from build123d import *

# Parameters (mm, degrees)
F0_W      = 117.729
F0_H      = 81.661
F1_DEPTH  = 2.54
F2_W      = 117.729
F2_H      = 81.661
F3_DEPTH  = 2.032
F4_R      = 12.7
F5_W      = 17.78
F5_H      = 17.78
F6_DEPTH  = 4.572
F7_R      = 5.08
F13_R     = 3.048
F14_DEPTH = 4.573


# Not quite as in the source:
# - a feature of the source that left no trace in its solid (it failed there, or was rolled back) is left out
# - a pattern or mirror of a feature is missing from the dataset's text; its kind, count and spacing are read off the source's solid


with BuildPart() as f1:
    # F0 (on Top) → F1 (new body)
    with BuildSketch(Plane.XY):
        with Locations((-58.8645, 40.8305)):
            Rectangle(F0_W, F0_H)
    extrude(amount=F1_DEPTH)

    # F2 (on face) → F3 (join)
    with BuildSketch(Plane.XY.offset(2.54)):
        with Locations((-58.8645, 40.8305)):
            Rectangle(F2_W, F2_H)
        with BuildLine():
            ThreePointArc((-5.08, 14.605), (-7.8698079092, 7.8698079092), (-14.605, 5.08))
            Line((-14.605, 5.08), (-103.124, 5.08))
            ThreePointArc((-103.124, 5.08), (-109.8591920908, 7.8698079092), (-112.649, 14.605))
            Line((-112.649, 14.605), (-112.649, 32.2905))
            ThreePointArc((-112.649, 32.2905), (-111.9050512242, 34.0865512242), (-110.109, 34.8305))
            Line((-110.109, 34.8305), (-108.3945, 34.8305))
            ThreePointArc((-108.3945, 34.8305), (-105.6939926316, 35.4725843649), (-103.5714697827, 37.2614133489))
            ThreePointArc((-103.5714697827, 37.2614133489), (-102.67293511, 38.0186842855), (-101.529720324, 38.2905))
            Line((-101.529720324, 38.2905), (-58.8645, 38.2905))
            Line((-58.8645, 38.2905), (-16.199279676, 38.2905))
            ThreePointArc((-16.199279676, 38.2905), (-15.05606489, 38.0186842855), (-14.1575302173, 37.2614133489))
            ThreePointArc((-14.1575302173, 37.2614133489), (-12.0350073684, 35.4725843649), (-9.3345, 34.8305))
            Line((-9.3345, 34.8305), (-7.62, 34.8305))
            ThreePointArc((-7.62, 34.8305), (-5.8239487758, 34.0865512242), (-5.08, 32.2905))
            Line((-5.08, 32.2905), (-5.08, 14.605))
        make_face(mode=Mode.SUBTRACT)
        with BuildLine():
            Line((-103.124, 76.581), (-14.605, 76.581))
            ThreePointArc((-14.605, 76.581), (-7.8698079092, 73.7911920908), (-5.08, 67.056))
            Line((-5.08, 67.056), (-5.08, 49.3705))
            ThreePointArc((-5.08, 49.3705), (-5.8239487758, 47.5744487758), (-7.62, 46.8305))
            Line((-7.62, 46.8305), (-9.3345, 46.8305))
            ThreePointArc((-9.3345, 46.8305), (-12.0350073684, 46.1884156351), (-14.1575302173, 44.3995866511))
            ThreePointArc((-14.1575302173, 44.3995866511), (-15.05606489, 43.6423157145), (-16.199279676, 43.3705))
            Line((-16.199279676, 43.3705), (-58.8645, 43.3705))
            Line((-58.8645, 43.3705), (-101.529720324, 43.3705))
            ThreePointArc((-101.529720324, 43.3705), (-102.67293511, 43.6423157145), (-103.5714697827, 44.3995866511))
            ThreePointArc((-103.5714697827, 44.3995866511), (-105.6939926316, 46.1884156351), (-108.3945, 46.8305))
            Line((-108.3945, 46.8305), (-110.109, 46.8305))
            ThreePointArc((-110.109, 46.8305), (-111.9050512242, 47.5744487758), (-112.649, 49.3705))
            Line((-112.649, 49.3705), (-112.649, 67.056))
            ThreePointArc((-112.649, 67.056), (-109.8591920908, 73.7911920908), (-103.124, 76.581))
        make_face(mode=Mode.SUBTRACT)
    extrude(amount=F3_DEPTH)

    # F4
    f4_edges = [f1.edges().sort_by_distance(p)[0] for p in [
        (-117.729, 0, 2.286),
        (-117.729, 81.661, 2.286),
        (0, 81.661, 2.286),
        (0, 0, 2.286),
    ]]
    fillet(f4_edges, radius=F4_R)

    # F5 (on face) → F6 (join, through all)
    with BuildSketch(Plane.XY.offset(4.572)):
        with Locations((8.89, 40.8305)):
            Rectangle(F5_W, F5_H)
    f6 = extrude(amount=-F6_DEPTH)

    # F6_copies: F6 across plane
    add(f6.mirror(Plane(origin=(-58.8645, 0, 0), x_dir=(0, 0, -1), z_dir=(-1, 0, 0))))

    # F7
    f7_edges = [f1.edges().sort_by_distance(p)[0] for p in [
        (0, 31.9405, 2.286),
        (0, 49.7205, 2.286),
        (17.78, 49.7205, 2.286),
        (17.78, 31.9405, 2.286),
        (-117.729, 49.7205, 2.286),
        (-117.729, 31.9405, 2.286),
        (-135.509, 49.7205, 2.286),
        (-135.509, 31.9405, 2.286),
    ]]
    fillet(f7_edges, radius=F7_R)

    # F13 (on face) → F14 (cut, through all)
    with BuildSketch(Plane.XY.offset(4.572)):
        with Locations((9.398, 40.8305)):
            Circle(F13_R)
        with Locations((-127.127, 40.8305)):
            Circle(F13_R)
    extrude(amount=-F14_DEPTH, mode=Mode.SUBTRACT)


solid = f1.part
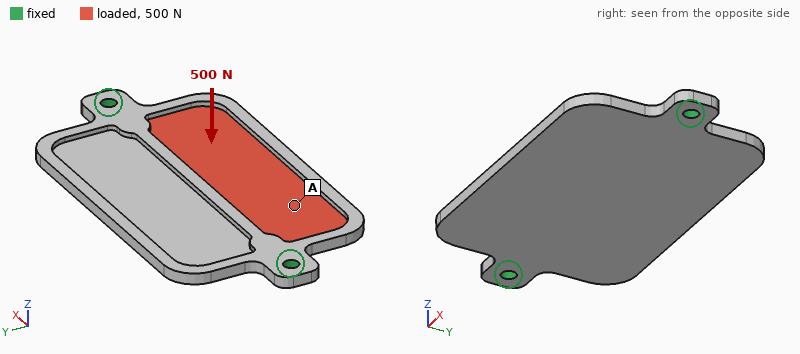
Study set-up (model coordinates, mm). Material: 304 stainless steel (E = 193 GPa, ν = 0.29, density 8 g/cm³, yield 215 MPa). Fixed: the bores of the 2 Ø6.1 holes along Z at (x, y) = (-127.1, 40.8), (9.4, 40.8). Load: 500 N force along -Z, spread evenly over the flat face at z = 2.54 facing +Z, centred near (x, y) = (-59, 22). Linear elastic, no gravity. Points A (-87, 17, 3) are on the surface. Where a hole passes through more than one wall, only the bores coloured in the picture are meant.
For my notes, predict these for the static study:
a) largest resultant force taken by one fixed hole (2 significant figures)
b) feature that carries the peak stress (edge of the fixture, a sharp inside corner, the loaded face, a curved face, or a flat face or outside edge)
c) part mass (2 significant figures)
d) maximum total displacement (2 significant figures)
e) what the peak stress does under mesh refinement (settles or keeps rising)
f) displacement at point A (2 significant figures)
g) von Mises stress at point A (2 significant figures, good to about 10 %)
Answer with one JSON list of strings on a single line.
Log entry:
["580 N", "edge of the fixture", "250 g", "0.27 mm", "keeps rising", "0.16 mm", "13 MPa"]
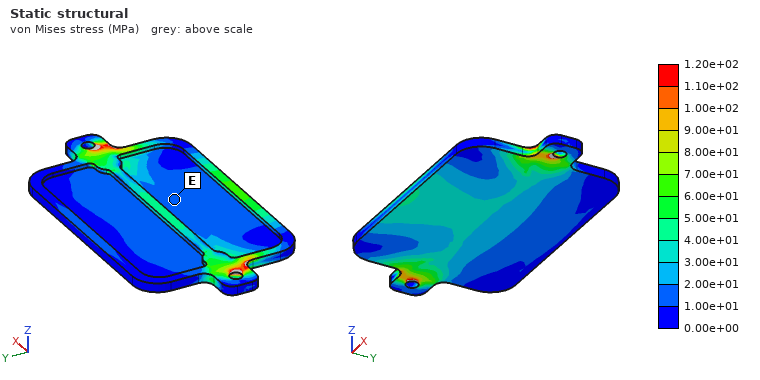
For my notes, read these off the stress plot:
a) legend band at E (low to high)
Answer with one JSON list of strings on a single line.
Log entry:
["1.00e+01 to 2.00e+01 MPa"]
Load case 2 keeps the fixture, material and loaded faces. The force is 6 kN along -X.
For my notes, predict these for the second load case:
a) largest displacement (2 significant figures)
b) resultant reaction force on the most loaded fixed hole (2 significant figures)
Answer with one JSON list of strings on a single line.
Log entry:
["39 µm", "3.1 kN"]
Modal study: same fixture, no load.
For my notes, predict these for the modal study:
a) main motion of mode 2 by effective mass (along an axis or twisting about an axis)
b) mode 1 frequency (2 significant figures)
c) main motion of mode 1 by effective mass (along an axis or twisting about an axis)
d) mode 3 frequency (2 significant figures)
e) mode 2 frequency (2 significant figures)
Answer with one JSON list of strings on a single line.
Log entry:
["along Z", "770 Hz", "twisting about X", "1700 Hz", "830 Hz"]
